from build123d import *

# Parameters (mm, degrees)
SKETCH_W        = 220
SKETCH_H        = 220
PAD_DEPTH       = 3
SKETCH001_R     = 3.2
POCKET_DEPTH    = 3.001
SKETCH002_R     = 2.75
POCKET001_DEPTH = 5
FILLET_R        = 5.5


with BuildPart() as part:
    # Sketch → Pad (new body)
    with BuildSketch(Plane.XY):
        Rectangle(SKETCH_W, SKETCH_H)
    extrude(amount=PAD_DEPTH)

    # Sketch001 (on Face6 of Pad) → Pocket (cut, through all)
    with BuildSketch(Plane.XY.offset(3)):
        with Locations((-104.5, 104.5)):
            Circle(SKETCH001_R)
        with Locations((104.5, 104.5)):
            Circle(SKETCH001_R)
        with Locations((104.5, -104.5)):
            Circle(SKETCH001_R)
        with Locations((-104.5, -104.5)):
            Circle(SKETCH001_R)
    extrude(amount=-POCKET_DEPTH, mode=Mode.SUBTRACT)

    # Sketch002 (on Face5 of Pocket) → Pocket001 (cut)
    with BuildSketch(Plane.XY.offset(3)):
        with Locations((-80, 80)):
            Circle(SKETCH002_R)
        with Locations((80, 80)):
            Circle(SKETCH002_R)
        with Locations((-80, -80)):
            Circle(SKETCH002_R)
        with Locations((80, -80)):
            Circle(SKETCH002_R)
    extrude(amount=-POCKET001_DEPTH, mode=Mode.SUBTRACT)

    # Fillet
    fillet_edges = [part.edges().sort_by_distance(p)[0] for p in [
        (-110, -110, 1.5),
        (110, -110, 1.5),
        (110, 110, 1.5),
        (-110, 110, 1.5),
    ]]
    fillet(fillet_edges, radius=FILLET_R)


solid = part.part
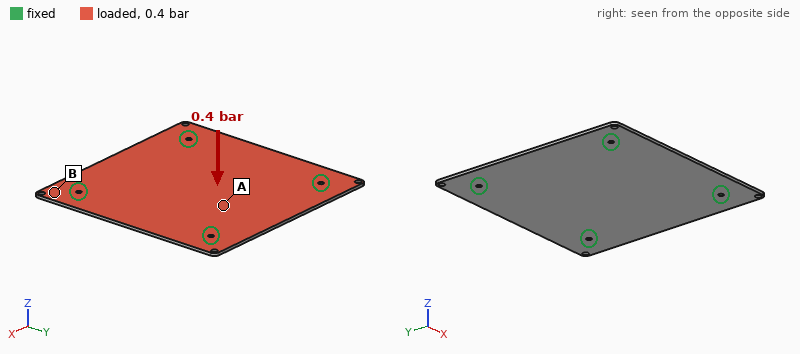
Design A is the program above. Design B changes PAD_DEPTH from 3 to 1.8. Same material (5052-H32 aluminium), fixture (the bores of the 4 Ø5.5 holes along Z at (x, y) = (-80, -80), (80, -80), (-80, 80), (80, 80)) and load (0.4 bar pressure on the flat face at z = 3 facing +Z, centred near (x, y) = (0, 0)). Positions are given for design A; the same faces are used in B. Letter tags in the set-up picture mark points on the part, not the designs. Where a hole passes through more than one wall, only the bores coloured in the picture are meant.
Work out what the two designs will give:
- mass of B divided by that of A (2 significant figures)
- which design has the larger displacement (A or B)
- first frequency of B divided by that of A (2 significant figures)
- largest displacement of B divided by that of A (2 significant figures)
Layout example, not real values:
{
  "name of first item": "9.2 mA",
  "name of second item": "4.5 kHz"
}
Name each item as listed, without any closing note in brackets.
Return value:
{
  "mass of B divided by that of A": "0.60",
  "which design has the larger displacement": "B",
  "first frequency of B divided by that of A": "0.61",
  "largest displacement of B divided by that of A": "4.5"
}
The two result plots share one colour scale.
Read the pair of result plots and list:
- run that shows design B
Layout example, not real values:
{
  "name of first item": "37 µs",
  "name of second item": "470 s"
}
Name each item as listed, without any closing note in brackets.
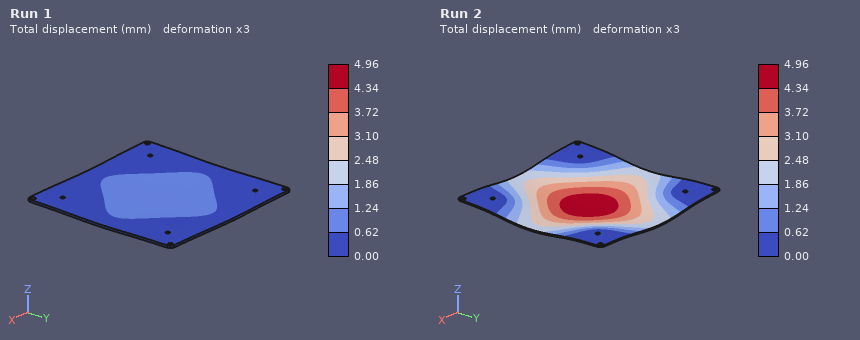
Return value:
{
  "run that shows design B": "Run 2"
}
